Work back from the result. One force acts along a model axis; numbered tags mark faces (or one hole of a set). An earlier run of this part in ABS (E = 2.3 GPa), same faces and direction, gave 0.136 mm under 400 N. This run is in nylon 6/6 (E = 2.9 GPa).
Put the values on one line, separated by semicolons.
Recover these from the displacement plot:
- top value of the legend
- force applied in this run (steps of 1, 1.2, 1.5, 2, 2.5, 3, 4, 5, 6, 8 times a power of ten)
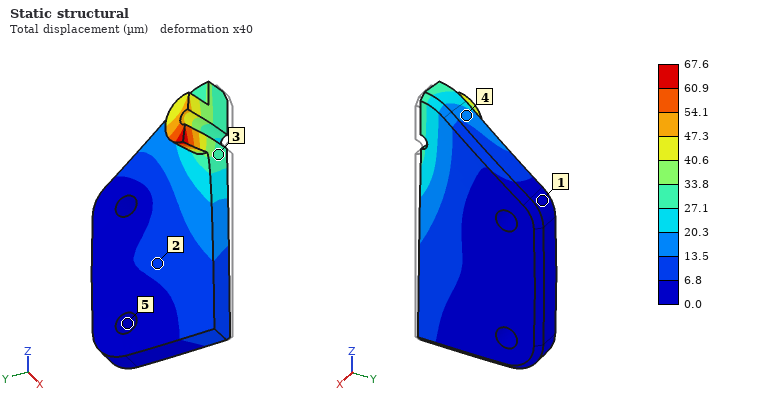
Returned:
67.6 µm; 250 N
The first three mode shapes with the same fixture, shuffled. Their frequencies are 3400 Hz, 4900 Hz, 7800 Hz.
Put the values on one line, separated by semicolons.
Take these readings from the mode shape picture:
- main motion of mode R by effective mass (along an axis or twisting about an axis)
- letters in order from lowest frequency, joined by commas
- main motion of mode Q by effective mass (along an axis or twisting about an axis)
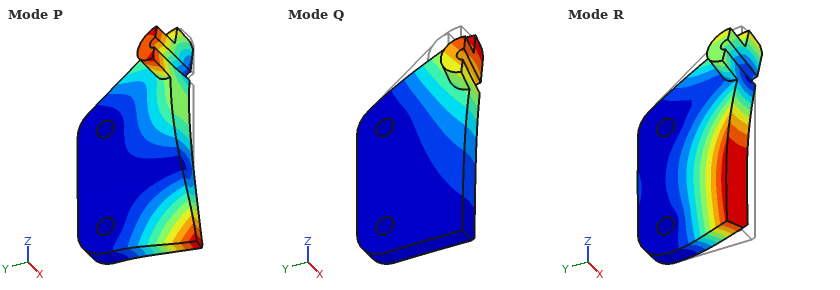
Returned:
along X; Q, R, P; along X
